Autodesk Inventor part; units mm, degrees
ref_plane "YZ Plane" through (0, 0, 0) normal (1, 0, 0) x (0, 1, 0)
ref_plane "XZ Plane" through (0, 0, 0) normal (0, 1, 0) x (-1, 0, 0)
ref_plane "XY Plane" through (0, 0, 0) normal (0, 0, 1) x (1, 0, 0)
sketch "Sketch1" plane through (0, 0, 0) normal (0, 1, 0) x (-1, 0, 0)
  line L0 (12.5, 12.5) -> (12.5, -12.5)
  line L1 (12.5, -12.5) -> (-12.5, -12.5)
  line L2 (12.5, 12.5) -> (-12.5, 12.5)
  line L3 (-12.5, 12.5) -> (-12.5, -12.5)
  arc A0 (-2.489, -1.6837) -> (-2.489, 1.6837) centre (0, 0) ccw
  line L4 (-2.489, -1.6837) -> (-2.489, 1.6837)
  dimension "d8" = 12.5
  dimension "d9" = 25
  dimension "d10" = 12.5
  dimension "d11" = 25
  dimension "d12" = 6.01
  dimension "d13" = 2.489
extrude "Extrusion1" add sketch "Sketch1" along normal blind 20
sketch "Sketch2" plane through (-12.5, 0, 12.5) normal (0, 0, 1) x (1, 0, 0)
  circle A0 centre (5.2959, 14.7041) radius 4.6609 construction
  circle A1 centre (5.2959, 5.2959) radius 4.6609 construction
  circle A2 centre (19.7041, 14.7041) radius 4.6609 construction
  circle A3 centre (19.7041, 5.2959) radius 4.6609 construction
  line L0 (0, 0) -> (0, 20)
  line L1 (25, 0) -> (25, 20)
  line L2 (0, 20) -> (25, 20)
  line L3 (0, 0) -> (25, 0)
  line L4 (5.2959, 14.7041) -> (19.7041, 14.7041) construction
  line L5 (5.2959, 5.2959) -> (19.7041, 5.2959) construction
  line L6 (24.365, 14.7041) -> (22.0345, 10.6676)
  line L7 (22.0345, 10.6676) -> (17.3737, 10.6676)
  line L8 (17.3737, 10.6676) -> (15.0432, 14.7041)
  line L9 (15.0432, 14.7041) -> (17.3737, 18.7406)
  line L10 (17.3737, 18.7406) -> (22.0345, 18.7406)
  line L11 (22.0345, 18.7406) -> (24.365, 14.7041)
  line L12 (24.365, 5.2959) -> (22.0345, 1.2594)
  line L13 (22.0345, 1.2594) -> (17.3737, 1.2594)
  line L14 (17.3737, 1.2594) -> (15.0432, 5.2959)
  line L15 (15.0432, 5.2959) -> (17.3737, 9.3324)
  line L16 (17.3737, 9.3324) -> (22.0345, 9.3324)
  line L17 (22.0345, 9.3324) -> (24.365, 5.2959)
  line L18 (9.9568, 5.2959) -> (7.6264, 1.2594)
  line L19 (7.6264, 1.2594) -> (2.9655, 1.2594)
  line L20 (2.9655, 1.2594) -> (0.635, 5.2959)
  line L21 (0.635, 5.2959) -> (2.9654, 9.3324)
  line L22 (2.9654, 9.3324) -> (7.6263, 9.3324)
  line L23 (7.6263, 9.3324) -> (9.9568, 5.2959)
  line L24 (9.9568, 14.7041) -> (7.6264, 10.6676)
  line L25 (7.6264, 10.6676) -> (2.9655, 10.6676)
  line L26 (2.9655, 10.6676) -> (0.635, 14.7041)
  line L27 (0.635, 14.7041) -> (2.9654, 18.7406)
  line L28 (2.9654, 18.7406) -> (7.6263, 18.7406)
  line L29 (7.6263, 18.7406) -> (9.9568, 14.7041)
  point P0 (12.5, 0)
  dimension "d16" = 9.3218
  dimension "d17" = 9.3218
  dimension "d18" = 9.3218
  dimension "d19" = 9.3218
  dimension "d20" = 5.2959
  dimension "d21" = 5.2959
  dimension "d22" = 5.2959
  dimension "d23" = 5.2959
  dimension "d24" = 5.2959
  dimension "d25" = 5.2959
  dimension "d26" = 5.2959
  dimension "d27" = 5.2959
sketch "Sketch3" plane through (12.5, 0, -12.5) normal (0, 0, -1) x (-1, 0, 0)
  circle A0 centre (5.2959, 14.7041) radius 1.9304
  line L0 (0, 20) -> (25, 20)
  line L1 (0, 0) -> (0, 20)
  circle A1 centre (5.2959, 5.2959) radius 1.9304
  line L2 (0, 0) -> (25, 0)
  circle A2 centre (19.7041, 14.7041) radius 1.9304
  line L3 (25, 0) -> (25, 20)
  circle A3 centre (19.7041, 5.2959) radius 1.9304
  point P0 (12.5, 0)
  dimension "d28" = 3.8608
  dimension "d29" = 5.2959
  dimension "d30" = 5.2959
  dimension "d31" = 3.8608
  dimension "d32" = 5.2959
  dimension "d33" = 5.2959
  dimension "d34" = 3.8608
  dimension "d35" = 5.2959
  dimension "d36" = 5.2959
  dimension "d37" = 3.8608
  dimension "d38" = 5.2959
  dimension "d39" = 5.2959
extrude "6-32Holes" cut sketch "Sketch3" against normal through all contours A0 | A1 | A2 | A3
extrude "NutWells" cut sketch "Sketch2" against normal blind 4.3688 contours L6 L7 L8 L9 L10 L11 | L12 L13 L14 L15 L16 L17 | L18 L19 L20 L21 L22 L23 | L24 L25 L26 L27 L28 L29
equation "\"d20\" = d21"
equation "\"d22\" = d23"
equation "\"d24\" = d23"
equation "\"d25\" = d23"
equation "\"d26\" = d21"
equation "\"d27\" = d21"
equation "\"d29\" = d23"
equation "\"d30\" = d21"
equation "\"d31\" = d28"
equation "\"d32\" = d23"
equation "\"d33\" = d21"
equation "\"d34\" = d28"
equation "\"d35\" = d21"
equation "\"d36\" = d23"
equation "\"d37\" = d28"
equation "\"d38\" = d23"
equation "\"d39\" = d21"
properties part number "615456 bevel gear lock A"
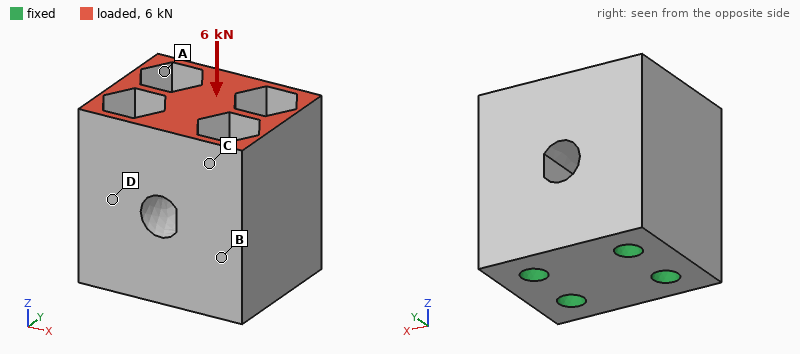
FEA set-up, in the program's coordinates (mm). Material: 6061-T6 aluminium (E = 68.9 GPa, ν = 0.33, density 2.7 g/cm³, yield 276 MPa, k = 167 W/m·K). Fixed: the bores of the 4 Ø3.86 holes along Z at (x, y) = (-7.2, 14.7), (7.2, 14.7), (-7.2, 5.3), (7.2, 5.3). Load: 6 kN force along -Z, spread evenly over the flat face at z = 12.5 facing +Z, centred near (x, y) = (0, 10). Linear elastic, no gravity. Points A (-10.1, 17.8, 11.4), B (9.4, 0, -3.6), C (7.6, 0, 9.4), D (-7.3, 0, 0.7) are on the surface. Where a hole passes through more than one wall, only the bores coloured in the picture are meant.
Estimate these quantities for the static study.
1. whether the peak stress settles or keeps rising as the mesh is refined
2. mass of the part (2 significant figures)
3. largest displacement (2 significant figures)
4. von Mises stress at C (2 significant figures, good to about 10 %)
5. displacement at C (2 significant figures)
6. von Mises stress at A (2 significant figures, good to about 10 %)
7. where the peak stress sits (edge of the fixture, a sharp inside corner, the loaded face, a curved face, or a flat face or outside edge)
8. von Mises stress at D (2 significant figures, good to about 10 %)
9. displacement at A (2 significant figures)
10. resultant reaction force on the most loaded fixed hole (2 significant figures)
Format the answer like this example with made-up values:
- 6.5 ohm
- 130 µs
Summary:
- keeps rising
- 27 g
- 4.1 µm
- 21 MPa
- 2.6 µm
- 24 MPa
- edge of the fixture
- 5.9 MPa
- 3.0 µm
- 1.6 kN
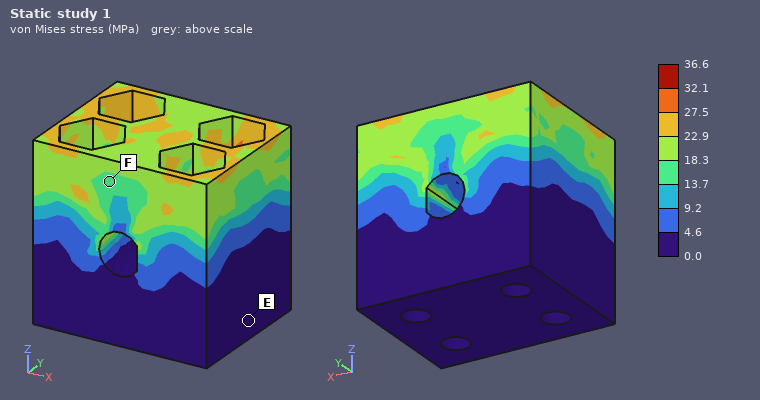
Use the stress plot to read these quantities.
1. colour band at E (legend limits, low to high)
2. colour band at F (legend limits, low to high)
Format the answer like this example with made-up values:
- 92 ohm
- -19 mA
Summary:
- 0.0 to 4.6 MPa
- 13.7 to 18.3 MPa
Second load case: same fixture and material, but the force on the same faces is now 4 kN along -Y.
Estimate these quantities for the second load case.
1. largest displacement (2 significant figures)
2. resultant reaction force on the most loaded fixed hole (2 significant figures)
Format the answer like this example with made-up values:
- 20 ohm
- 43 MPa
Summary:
- 16 µm
- 1.4 kN
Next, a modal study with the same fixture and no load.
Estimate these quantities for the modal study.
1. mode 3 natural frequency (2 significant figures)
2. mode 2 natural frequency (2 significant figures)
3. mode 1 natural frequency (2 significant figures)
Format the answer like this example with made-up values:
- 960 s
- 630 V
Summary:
- 84 kHz
- 84 kHz
- 70 kHz
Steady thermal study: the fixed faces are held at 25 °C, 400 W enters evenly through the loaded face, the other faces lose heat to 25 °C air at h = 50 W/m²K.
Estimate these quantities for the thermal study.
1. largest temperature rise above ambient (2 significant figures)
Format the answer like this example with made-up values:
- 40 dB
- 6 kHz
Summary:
- 70 K
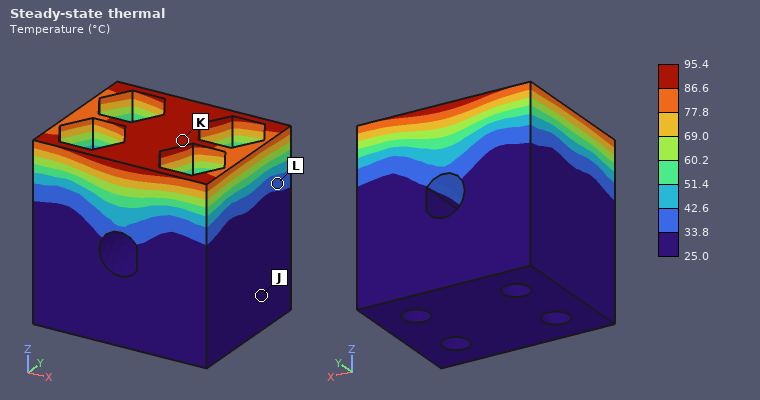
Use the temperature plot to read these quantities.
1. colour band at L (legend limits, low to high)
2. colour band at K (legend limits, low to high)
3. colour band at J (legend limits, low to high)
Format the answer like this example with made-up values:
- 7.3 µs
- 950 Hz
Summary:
- 33.8 to 42.6 °C
- 86.6 to 95.4 °C
- 25.0 to 33.8 °C
